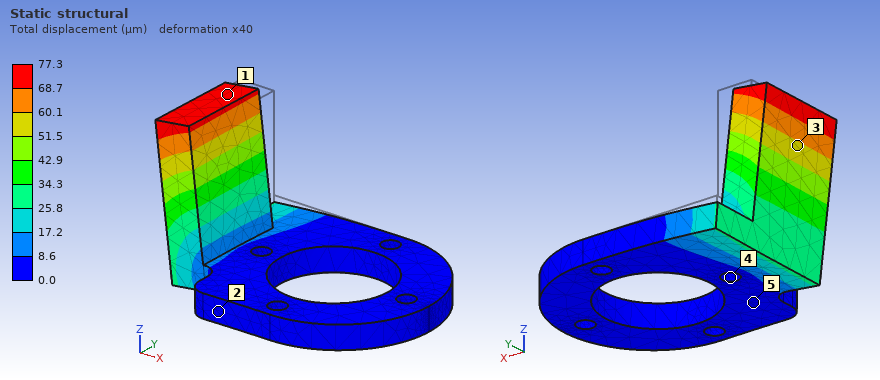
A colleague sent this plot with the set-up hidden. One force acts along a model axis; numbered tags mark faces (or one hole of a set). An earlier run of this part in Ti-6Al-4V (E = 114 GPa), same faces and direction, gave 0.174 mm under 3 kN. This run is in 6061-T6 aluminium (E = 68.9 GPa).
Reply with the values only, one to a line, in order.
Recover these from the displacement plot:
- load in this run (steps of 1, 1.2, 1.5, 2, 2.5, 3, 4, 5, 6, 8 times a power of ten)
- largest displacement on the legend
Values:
800 N
77.3 µm
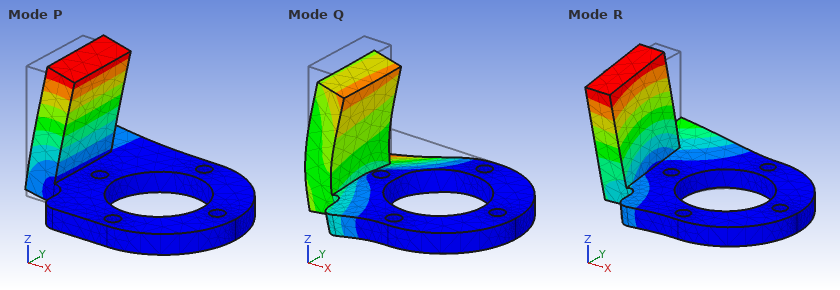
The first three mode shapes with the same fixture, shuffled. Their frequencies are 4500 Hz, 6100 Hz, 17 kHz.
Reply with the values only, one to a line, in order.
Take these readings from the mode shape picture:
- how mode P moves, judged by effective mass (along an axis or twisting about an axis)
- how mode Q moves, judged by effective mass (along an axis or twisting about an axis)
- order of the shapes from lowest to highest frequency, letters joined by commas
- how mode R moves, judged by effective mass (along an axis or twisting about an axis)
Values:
along X
along Z
P, R, Q
along Y
